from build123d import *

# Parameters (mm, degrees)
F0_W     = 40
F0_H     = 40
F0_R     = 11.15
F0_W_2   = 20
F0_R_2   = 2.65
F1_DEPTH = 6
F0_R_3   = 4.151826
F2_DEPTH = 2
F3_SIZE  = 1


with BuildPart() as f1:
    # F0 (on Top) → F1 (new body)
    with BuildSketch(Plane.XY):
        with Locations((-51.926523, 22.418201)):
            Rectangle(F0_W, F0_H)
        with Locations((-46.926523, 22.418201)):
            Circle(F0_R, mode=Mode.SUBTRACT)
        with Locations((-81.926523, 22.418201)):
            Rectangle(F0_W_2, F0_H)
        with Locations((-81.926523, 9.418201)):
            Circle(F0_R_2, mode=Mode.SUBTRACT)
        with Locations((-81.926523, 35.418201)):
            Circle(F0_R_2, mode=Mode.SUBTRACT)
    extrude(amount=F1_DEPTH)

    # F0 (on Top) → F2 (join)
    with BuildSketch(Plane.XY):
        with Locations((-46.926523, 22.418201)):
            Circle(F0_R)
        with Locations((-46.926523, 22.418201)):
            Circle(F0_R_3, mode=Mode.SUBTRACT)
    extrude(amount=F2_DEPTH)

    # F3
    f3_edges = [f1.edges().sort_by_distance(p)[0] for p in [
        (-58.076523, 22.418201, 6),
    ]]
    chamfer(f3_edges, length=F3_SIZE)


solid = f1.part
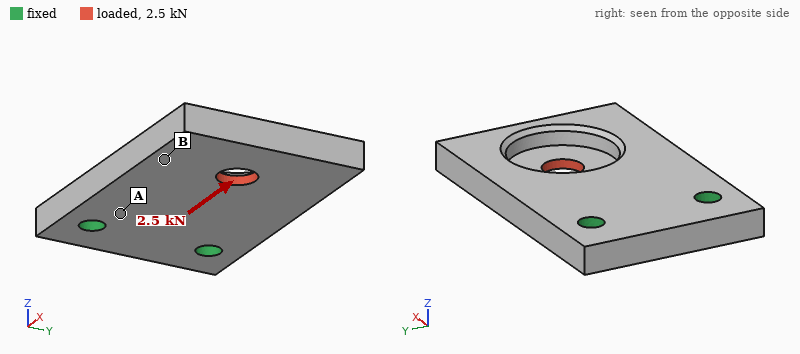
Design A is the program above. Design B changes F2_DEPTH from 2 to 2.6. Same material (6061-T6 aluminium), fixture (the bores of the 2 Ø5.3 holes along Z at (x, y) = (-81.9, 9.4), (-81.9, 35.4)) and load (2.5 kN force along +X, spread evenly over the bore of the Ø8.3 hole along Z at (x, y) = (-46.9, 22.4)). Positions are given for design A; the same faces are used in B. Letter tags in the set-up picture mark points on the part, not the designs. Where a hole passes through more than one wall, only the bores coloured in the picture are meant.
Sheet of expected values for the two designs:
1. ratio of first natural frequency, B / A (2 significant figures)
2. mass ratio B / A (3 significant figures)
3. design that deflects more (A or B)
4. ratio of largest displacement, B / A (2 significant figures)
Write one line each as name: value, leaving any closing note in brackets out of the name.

ratio of first natural frequency, B / A: 0.99
mass ratio B / A: 1.02
design that deflects more: A
ratio of largest displacement, B / A: 0.84
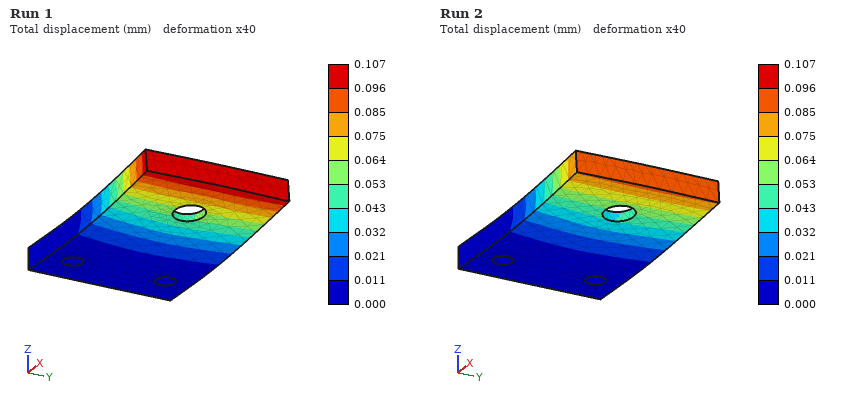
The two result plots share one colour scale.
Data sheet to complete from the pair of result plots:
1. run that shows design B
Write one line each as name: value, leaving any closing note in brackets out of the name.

run that shows design B: Run 2
